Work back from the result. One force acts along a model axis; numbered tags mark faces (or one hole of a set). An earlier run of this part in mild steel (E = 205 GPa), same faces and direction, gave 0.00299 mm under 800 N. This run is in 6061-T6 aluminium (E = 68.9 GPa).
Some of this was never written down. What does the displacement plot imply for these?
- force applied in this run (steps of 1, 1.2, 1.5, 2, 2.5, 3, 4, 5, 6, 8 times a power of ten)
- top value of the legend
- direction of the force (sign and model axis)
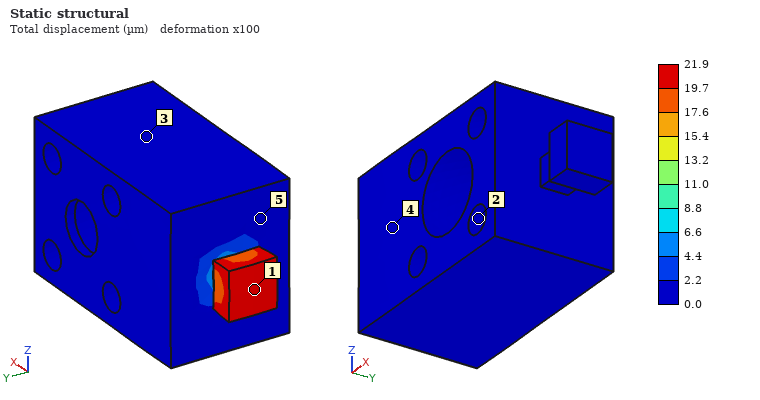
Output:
2 kN
21.9 µm
+X
